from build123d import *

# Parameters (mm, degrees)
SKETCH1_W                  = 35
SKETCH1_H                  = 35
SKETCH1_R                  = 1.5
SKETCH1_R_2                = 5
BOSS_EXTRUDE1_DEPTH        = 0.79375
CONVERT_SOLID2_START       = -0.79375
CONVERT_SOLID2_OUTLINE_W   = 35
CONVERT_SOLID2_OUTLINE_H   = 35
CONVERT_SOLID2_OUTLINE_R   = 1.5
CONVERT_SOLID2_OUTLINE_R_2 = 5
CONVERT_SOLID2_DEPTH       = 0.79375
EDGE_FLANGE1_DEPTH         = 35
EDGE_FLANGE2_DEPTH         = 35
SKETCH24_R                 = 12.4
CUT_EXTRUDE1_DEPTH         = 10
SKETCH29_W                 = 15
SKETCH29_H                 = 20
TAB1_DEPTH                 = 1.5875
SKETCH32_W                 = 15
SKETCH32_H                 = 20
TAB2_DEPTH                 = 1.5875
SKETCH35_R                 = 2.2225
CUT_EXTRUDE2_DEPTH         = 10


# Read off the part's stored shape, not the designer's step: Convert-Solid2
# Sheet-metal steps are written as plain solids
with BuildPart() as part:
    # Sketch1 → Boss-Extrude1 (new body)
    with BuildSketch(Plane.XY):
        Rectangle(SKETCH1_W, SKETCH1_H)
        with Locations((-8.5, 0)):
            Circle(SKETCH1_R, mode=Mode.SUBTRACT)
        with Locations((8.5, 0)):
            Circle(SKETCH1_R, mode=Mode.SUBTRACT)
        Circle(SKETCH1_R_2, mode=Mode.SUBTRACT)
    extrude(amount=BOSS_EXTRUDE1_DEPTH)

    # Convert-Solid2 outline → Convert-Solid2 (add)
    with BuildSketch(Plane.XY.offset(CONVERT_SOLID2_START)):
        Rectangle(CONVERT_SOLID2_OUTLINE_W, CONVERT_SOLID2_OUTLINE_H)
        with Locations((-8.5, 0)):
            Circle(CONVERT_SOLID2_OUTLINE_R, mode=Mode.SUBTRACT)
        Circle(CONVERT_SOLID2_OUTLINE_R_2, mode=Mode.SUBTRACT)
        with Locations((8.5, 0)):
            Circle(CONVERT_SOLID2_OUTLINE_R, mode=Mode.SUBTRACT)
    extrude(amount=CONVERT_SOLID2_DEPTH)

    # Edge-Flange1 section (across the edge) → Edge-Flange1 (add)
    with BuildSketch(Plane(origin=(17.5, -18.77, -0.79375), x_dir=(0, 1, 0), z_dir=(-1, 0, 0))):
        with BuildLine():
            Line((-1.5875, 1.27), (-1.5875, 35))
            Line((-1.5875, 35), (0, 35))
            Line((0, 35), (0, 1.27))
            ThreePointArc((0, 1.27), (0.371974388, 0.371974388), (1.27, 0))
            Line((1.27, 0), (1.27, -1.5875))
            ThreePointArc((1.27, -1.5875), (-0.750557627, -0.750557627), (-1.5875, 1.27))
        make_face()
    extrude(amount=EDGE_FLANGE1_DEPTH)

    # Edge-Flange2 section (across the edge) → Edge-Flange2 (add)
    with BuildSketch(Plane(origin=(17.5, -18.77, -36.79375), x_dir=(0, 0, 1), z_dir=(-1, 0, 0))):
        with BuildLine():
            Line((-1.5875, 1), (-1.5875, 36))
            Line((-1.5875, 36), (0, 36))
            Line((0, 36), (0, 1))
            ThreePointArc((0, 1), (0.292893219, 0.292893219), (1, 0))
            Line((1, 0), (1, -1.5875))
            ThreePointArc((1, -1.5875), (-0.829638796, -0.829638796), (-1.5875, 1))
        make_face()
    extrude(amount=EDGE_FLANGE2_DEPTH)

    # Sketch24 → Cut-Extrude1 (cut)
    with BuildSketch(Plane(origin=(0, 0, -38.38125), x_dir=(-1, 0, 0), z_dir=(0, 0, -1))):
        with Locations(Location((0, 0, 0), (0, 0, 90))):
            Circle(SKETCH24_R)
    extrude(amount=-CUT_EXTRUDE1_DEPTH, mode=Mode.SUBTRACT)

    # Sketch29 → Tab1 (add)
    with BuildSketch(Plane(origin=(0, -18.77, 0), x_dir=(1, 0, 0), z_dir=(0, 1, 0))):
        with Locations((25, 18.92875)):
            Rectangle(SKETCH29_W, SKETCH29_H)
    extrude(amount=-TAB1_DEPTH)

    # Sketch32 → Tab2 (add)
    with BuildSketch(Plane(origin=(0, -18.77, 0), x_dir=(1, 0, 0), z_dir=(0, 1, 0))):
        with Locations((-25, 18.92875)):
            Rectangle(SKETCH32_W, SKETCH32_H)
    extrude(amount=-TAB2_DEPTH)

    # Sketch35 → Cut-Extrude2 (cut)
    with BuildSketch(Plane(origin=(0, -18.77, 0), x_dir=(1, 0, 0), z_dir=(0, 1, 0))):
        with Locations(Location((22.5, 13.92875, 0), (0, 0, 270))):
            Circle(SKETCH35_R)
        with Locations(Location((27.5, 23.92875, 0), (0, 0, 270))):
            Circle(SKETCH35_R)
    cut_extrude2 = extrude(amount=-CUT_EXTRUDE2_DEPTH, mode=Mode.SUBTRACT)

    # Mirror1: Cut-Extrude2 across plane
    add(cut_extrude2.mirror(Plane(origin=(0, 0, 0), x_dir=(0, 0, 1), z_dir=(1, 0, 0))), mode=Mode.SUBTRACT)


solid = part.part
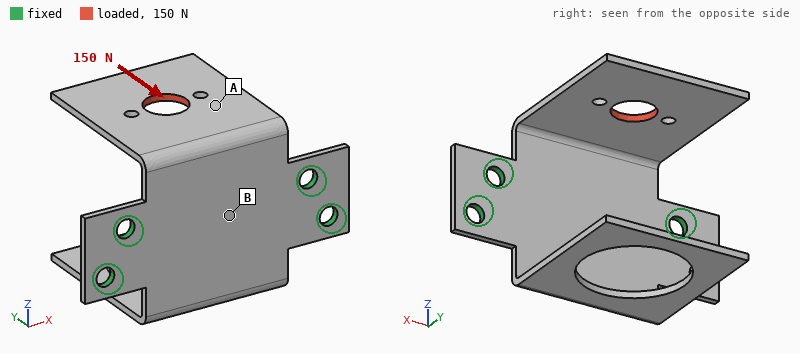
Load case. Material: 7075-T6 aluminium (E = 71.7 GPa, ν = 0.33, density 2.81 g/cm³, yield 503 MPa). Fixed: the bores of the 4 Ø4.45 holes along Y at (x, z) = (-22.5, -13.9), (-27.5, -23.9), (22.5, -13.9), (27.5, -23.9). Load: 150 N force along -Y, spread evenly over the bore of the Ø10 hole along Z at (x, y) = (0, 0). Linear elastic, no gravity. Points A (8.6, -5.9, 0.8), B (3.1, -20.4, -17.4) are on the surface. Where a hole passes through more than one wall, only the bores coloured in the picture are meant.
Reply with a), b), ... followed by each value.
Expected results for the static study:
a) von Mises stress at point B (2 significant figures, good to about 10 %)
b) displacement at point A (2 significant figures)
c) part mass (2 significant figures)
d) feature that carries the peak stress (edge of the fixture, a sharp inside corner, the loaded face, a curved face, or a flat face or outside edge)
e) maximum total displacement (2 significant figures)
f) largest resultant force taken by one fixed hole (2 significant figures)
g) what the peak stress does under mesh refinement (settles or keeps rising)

a) 40 MPa
b) 0.43 mm
c) 17 g
d) edge of the fixture
e) 0.90 mm
f) 110 N
g) keeps rising
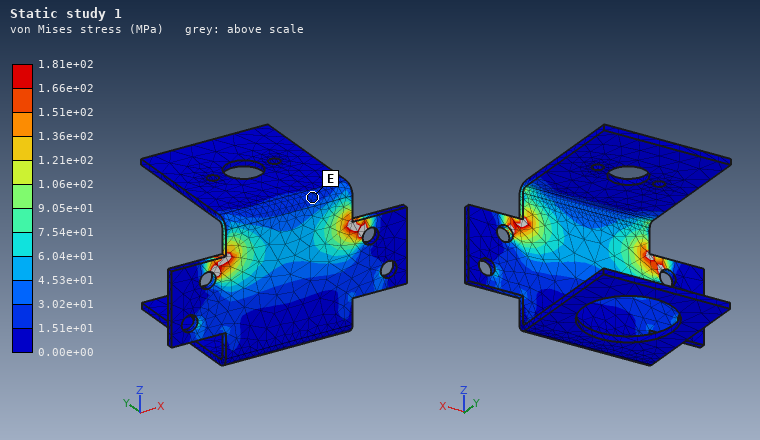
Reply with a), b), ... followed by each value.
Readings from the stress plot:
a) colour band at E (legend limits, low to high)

a) 1.51e+01 to 3.02e+01 MPa
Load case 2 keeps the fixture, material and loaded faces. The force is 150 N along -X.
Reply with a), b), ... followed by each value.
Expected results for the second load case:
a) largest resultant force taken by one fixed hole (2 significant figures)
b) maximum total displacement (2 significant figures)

a) 120 N
b) 0.46 mm
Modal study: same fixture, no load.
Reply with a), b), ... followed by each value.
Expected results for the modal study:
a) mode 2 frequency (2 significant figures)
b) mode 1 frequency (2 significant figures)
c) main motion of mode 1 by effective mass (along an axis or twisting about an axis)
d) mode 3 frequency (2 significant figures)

a) 610 Hz
b) 570 Hz
c) along Z
d) 1400 Hz
